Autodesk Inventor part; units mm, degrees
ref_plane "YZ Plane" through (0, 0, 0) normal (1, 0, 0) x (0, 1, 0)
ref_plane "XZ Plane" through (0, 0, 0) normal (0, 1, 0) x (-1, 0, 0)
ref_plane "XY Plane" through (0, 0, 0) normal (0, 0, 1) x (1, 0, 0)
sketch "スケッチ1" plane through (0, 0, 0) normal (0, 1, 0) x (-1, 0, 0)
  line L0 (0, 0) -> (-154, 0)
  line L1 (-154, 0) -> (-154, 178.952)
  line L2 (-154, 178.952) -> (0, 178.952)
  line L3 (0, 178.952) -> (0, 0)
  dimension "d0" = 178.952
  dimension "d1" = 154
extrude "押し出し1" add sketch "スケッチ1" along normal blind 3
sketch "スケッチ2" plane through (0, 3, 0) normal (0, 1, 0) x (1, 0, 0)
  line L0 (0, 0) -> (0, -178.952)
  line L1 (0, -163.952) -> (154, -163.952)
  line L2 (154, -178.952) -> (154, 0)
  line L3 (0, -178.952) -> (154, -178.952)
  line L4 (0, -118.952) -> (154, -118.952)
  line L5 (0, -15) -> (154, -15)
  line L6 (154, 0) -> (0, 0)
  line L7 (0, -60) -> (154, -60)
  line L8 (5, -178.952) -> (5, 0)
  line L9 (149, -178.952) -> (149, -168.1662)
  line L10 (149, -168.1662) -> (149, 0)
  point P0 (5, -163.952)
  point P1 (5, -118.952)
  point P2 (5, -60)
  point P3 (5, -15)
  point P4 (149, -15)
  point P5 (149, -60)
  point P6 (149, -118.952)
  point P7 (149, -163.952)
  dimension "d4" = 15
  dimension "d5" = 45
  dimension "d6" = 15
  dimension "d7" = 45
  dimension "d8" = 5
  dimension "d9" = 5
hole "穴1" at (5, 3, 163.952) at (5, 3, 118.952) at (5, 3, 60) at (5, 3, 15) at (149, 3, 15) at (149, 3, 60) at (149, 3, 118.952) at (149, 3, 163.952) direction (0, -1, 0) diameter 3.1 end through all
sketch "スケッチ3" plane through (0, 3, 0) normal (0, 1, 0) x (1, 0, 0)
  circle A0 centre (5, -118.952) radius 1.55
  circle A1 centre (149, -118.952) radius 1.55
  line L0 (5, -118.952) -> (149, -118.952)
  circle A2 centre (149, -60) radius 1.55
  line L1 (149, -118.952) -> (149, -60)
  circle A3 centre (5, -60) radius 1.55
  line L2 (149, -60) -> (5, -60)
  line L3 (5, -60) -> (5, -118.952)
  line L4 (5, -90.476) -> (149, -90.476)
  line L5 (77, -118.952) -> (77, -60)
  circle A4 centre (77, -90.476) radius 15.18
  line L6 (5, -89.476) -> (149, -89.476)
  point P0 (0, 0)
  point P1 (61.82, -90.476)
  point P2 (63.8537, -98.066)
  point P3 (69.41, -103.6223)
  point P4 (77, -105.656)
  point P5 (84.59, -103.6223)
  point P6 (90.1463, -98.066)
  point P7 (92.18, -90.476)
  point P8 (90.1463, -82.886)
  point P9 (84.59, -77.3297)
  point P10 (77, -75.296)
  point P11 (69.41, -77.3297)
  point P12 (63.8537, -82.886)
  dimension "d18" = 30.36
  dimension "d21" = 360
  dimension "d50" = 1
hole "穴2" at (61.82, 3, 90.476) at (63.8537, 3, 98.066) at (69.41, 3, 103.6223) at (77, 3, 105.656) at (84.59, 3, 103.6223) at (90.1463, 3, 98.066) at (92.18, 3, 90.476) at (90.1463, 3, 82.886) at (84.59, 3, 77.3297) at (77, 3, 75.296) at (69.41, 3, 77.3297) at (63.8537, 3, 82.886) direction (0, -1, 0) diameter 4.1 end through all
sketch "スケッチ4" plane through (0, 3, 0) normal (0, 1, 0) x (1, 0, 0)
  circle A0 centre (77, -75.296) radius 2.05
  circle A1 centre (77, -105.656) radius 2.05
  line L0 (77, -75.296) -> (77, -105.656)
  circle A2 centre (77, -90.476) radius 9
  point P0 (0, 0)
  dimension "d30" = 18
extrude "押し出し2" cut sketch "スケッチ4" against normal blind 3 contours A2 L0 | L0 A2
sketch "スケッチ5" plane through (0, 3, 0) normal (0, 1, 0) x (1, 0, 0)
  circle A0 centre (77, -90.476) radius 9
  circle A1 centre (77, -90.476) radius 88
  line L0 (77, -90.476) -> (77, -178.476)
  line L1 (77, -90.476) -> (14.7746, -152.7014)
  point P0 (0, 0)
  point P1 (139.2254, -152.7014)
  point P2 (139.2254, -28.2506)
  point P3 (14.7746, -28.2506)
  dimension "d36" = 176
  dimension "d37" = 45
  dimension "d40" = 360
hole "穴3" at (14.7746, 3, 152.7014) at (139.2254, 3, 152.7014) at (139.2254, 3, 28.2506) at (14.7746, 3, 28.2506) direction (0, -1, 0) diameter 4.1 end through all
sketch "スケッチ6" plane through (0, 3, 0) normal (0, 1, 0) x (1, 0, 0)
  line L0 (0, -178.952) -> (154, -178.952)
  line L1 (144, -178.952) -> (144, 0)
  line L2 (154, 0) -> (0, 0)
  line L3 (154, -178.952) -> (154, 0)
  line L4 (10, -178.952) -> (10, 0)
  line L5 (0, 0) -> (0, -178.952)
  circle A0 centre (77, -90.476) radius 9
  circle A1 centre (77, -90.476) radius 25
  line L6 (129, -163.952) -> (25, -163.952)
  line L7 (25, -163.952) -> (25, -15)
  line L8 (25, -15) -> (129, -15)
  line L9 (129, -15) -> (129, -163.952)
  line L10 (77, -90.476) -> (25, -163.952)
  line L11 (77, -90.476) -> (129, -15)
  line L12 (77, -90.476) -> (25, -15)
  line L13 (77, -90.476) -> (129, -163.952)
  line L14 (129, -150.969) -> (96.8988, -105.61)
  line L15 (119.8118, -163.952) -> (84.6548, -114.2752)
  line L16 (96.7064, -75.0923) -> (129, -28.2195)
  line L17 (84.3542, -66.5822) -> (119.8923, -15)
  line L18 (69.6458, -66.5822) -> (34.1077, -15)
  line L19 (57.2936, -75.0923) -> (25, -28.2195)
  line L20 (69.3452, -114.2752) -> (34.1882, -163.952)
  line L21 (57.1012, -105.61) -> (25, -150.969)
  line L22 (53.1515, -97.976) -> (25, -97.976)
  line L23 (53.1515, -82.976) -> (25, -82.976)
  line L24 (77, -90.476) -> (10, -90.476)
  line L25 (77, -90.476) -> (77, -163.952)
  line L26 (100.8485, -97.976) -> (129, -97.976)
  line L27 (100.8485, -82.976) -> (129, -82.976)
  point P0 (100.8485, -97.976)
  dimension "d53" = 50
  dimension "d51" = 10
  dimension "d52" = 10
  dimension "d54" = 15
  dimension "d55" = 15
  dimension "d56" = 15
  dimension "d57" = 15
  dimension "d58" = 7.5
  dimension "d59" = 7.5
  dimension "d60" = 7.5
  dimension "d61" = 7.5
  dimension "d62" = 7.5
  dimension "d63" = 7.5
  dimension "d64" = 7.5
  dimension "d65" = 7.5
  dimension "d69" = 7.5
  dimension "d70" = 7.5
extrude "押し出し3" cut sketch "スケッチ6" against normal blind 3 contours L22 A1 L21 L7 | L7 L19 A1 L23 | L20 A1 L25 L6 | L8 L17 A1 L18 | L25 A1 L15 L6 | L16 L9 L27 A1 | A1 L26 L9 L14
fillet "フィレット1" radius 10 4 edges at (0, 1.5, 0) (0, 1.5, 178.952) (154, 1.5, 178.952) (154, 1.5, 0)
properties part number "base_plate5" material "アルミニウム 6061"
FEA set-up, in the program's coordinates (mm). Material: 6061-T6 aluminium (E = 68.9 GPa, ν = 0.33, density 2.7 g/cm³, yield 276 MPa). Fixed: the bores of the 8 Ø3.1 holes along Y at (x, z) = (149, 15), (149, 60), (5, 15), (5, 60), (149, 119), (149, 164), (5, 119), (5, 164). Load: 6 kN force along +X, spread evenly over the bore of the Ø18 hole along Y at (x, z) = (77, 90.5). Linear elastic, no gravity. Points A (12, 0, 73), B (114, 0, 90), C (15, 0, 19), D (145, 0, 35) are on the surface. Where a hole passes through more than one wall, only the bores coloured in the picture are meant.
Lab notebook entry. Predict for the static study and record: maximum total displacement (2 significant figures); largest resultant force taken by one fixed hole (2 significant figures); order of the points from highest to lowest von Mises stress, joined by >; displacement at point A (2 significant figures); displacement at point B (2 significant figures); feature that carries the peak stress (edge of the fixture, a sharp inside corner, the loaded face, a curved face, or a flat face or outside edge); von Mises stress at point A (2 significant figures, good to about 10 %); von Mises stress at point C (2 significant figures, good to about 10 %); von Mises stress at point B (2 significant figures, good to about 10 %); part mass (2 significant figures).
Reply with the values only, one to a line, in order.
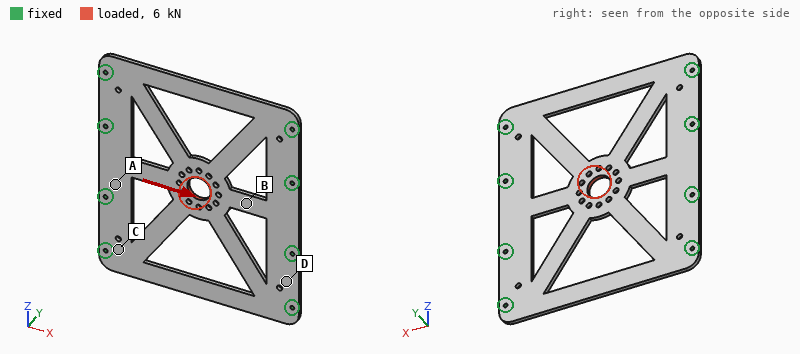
54 µm
1.2 kN
B > A > C > D
13 µm
34 µm
a curved face
32 MPa
17 MPa
42 MPa
150 g
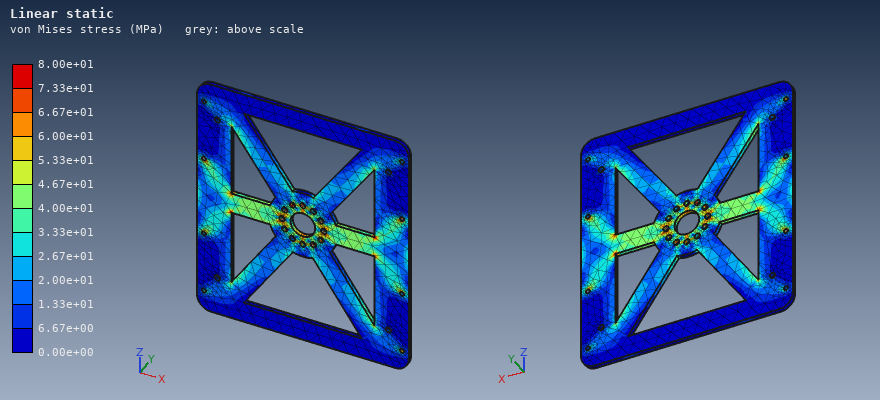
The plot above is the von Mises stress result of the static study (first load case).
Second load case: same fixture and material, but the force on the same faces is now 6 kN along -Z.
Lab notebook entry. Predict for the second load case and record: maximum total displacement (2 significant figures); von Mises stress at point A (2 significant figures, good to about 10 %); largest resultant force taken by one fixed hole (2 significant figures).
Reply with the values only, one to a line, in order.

71 µm
11 MPa
1.0 kN
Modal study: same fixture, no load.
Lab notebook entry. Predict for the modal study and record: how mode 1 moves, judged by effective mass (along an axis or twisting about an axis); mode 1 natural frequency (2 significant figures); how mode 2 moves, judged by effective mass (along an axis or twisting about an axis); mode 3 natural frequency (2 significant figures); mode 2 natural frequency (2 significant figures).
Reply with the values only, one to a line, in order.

along Y
660 Hz
twisting about X
950 Hz
860 Hz
